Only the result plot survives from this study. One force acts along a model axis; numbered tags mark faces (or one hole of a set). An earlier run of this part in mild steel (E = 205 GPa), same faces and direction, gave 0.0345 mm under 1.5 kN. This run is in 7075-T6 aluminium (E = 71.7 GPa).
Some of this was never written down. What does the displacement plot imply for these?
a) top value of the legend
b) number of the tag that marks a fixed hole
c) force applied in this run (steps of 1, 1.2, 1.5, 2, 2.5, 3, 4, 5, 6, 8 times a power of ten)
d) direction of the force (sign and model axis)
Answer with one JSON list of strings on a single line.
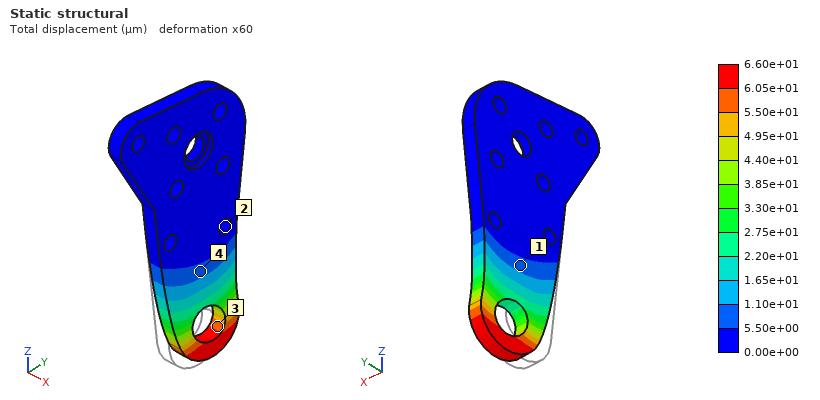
["6.60e+01 µm", "2", "1 kN", "+Y"]
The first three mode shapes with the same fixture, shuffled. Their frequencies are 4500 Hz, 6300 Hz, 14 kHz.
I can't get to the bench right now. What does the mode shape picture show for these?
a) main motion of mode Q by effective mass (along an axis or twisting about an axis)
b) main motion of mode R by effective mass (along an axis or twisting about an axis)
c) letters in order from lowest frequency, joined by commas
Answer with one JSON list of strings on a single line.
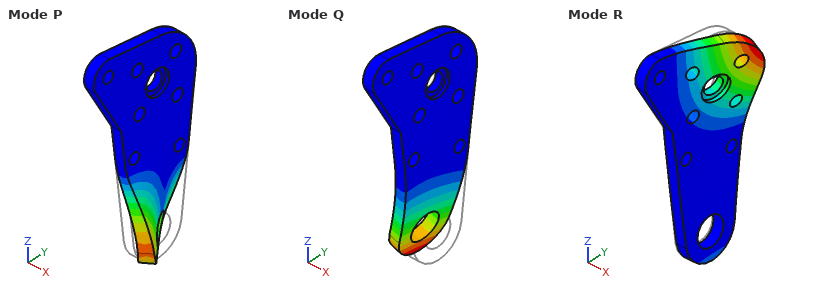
["along X", "along X", "Q, R, P"]
